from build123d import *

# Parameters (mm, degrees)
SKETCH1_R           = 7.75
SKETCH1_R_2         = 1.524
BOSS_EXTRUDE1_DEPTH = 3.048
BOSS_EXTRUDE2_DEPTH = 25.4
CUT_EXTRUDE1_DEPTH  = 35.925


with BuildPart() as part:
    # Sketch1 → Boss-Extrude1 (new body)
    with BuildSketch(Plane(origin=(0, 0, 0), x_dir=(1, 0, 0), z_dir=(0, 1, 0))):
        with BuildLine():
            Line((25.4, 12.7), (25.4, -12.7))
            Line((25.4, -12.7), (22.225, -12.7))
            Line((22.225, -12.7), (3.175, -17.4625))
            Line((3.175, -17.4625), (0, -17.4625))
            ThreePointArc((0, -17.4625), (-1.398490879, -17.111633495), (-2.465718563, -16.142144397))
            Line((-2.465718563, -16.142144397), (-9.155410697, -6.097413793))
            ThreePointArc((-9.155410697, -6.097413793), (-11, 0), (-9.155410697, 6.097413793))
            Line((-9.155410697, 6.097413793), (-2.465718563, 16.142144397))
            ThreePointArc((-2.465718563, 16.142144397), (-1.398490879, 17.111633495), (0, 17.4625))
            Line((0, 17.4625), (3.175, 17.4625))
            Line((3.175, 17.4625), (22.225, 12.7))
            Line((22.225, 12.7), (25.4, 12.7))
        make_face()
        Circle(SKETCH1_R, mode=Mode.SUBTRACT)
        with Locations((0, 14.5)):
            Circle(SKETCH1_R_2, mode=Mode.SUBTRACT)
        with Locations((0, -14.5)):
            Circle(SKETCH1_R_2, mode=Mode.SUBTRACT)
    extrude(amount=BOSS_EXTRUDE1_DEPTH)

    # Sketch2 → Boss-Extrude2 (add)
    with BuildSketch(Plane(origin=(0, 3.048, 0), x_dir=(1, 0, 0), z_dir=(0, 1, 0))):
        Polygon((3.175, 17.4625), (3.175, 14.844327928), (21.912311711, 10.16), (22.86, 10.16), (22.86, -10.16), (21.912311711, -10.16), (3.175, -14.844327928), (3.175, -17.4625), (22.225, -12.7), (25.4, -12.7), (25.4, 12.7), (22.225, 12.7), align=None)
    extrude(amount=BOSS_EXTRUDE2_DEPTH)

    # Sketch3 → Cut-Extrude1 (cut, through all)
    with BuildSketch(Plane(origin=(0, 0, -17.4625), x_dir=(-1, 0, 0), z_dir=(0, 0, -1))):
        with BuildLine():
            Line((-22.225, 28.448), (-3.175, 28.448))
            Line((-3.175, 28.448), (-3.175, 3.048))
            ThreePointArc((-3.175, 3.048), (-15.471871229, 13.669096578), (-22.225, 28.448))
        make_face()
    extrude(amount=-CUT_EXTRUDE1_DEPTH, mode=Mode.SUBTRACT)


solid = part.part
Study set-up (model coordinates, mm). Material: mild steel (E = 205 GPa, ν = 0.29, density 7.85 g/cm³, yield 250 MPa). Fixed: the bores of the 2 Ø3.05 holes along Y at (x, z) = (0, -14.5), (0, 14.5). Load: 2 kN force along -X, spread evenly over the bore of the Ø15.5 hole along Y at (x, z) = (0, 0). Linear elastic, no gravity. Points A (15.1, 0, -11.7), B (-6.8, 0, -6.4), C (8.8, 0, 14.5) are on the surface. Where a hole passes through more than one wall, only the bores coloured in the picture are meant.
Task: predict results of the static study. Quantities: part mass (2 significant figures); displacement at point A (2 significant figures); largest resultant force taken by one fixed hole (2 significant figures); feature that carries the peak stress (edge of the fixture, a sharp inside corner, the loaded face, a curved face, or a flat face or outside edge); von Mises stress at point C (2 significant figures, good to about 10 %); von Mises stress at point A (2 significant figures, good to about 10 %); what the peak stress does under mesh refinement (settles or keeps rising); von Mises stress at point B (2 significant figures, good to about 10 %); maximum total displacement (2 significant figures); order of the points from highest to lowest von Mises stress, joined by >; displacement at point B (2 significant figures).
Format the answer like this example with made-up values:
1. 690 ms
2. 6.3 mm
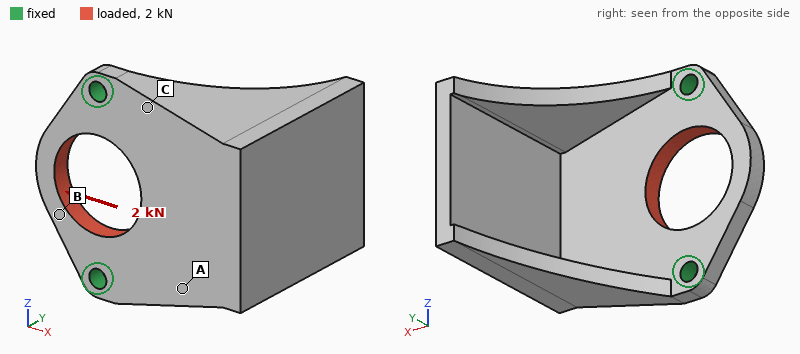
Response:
1. 40 g
2. 1.8 µm
3. 1.0 kN
4. edge of the fixture
5. 23 MPa
6. 9.5 MPa
7. keeps rising
8. 41 MPa
9. 4.9 µm
10. B > C > A
11. 3.5 µm
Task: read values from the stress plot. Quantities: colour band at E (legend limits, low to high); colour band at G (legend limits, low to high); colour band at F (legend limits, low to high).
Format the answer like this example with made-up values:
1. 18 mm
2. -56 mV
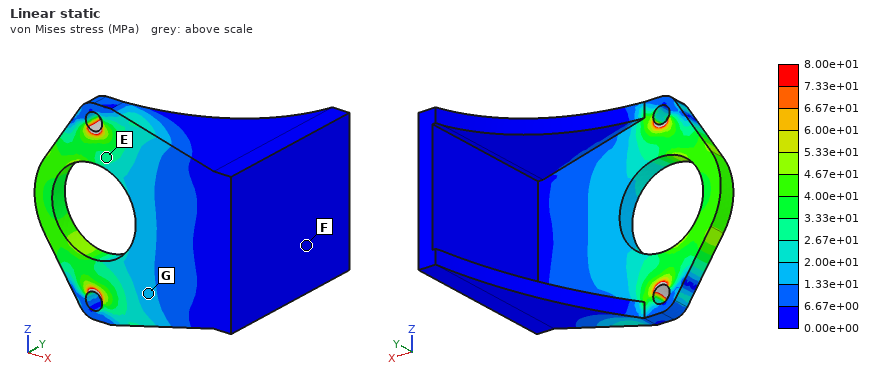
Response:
1. 2.67e+01 to 3.33e+01 MPa
2. 1.33e+01 to 2.00e+01 MPa
3. 0.00e+00 to 6.67e+00 MPa
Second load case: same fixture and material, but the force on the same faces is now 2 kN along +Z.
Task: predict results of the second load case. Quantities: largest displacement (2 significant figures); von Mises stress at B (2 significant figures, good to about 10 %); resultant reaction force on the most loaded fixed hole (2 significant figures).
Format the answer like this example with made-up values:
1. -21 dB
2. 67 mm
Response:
1. 4.5 µm
2. 37 MPa
3. 1.0 kN
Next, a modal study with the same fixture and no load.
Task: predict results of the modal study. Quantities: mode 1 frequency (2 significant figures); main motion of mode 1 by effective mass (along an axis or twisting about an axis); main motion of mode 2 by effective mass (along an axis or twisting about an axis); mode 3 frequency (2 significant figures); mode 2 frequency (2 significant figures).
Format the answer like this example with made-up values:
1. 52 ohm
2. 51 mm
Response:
1. 1600 Hz
2. along Y
3. along Z
4. 10 kHz
5. 3700 Hz
